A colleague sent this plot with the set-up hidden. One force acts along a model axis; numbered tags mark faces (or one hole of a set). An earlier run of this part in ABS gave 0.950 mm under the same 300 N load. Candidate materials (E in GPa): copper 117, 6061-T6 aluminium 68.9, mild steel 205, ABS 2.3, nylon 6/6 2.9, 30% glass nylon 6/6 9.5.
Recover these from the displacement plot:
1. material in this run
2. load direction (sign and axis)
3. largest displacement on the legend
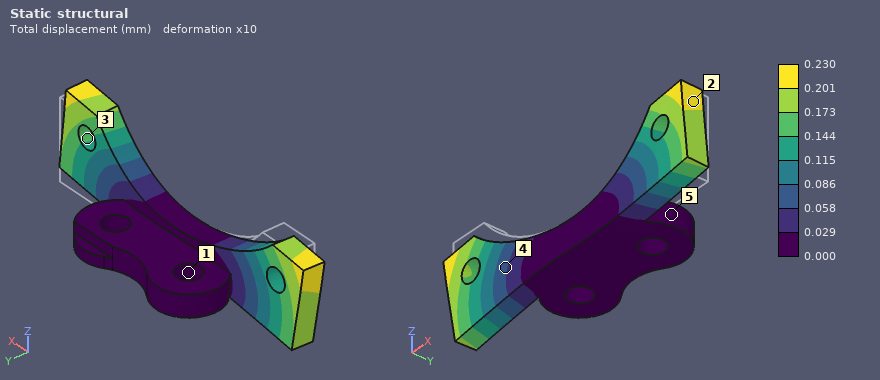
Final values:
30% glass nylon 6/6
-X
0.230 mm
